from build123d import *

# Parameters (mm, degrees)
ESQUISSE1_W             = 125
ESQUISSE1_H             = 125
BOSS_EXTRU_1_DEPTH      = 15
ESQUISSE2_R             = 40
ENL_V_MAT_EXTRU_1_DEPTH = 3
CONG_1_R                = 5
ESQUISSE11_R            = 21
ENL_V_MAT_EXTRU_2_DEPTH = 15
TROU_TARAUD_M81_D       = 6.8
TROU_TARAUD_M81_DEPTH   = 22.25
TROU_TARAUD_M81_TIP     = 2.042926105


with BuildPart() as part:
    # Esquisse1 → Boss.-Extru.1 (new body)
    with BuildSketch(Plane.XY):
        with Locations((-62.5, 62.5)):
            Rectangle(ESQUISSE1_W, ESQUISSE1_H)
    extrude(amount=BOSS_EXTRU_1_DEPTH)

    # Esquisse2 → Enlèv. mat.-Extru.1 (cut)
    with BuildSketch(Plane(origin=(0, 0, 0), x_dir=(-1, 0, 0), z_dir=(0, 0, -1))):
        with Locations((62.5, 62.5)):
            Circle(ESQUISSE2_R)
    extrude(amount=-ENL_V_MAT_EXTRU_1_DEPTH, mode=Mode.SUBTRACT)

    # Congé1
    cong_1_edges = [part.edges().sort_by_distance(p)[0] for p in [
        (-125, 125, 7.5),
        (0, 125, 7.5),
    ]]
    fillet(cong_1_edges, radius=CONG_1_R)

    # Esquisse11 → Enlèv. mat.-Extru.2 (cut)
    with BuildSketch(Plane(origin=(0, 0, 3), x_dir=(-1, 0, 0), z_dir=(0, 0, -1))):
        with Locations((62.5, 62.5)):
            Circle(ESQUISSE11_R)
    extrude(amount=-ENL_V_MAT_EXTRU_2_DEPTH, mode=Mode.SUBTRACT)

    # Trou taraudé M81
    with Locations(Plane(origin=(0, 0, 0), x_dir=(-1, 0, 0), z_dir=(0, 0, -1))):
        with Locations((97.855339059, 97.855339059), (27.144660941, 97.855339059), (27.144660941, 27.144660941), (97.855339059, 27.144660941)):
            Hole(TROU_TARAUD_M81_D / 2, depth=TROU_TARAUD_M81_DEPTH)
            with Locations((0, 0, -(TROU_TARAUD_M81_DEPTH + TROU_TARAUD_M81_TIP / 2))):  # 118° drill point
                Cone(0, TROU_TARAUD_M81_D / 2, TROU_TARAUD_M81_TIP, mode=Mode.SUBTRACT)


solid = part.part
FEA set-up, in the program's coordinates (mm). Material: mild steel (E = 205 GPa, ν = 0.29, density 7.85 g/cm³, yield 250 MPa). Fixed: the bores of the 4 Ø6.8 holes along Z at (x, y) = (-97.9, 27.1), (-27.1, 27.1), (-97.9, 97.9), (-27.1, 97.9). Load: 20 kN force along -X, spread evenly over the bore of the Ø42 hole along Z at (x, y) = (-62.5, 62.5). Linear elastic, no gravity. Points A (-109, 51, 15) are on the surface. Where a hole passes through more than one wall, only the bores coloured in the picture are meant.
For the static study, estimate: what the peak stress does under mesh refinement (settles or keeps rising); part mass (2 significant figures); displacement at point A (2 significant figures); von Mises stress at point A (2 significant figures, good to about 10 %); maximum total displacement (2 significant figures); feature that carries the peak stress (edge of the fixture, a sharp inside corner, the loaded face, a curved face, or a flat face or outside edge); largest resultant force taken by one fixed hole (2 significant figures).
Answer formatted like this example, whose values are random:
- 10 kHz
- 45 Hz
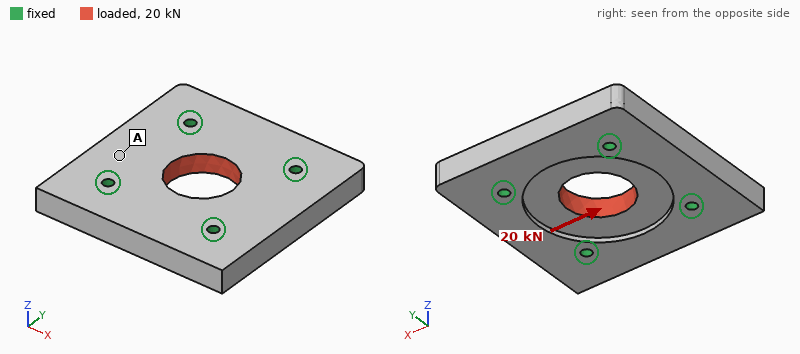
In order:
- keeps rising
- 1.6 kg
- 2.1 µm
- 7.5 MPa
- 3.5 µm
- edge of the fixture
- 5.1 kN
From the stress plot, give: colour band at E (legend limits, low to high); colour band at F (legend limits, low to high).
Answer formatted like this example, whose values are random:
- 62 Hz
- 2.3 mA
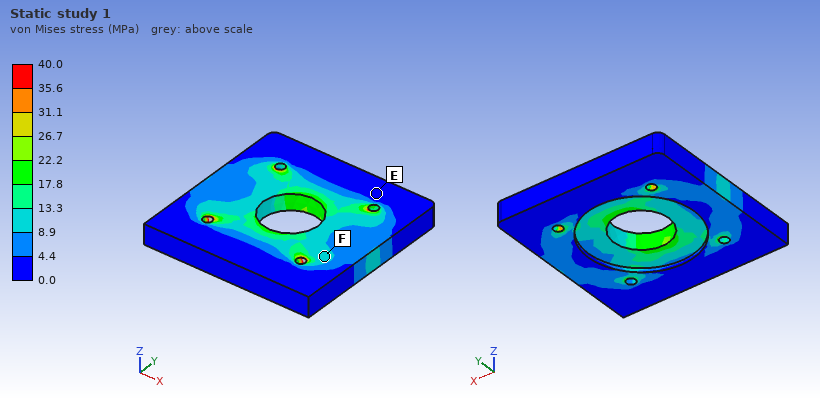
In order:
- 0.0 to 4.4 MPa
- 8.9 to 13.3 MPa
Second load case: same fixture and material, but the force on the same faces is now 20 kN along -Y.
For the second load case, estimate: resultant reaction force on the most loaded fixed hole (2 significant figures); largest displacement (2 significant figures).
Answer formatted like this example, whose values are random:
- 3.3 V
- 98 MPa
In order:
- 5.1 kN
- 3.5 µm
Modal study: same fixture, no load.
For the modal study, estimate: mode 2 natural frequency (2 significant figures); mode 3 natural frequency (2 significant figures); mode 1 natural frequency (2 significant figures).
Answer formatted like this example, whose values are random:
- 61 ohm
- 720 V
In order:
- 9100 Hz
- 9100 Hz
- 8100 Hz
